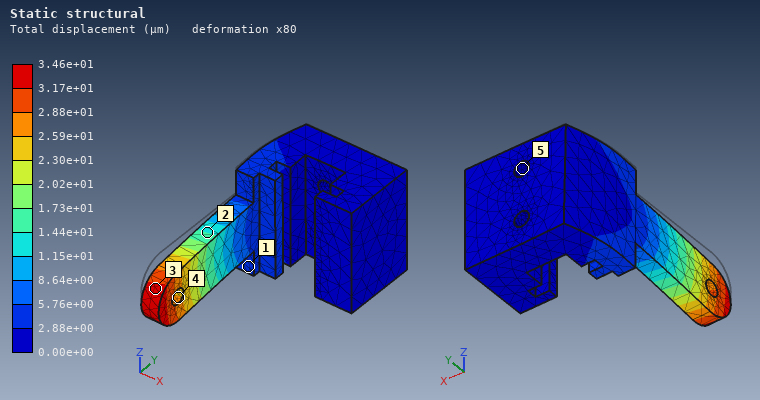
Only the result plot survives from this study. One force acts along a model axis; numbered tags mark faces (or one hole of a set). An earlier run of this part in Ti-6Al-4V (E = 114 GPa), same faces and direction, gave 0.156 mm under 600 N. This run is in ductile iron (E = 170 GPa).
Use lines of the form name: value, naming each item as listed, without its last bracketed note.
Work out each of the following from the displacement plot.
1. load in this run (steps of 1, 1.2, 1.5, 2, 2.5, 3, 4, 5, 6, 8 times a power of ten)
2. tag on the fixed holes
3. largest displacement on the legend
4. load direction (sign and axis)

load in this run: 200 N
tag on the fixed holes: 5
largest displacement on the legend: 3.46e+01 µm
load direction: -Z
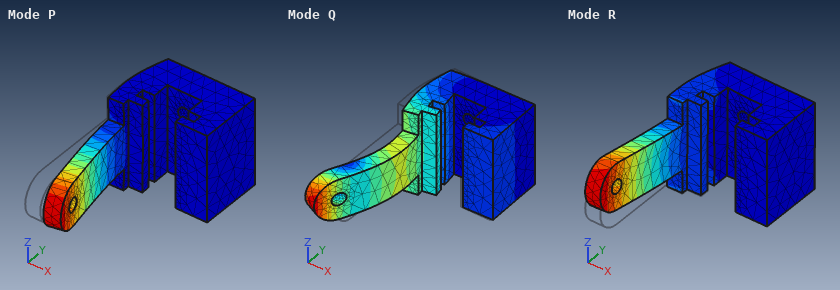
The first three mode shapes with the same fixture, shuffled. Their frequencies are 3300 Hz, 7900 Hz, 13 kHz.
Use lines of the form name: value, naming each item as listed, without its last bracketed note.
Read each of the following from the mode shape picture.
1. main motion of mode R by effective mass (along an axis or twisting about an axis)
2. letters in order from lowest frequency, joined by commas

main motion of mode R by effective mass: along Z
letters in order from lowest frequency, joined by commas: P, R, Q
